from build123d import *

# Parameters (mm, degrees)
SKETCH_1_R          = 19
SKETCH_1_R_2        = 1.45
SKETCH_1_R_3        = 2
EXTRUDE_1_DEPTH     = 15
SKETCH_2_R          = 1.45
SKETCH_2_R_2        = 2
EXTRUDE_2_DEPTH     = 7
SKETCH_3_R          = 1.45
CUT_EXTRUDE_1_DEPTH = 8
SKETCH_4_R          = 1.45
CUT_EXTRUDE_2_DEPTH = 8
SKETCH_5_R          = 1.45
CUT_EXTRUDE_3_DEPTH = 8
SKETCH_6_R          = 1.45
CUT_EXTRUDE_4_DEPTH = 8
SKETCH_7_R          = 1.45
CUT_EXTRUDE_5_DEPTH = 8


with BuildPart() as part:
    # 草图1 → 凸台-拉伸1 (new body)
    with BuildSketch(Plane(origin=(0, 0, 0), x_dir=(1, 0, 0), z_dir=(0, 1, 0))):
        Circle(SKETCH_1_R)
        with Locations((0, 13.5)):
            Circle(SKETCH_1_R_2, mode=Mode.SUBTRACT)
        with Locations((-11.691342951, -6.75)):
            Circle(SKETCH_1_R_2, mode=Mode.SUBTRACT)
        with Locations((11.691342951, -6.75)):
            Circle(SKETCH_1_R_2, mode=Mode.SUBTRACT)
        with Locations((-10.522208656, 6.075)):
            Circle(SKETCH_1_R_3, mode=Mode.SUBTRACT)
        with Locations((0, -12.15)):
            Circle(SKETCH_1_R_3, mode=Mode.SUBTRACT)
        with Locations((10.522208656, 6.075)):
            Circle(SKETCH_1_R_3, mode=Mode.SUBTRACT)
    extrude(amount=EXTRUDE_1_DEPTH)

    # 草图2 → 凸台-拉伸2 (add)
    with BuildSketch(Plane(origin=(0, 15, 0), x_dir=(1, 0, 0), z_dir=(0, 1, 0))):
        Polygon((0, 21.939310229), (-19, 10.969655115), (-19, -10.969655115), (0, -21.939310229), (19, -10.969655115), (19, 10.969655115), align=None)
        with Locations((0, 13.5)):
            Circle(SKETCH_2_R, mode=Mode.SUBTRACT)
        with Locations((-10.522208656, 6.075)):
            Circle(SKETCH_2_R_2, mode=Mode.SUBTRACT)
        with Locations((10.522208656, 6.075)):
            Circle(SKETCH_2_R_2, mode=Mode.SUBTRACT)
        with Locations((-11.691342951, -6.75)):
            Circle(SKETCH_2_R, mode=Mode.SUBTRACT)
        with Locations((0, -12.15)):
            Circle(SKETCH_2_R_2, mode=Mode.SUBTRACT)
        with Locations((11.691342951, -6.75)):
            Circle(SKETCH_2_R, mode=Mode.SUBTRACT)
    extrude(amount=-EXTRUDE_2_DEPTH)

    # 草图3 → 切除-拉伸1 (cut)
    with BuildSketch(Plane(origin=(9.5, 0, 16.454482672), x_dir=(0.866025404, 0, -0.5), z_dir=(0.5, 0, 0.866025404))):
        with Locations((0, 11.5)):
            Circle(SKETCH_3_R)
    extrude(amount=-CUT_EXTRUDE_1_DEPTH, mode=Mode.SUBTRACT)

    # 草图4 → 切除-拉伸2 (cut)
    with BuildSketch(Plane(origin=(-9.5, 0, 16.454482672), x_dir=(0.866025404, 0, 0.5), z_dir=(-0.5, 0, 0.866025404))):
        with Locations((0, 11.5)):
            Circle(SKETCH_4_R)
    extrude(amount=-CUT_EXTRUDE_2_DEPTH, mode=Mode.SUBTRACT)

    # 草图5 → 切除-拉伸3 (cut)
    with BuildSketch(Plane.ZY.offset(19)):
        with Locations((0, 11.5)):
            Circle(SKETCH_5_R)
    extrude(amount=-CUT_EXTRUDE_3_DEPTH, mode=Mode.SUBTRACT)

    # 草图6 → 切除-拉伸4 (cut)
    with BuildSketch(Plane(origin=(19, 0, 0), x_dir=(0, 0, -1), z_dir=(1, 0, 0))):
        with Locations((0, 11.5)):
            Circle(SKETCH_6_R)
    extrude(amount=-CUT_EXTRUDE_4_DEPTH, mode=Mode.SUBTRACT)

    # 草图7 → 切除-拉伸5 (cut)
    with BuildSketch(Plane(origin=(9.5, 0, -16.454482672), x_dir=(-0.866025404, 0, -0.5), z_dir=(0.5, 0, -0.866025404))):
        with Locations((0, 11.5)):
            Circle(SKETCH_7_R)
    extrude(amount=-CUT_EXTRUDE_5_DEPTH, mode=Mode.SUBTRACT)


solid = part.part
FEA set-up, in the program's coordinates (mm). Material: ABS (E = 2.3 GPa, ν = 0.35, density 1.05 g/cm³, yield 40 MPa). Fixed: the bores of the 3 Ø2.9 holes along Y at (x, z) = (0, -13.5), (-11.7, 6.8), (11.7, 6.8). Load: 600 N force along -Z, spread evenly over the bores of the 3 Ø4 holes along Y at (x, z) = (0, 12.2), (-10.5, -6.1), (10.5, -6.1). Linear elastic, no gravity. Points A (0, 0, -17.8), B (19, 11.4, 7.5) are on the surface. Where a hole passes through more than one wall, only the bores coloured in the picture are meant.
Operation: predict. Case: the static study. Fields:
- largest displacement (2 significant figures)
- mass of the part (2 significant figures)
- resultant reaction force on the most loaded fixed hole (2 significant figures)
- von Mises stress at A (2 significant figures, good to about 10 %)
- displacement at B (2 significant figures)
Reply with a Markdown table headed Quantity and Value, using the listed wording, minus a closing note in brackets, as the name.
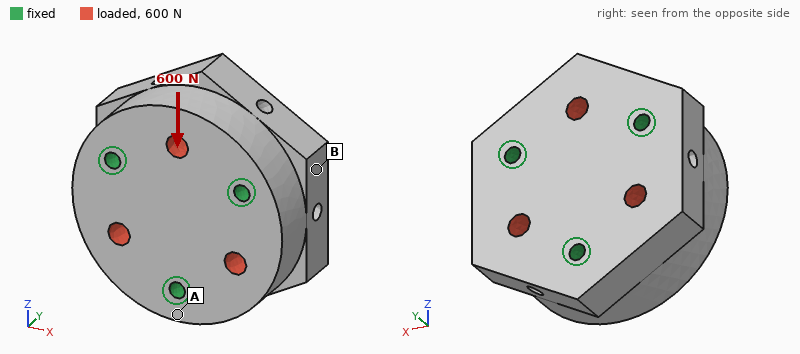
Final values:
| Quantity | Value |
|---|---|
| largest displacement | 8.4 µm |
| mass of the part | 18 g |
| resultant reaction force on the most loaded fixed hole | 210 N |
| von Mises stress at A | 0.79 MPa |
| displacement at B | 2.0 µm |
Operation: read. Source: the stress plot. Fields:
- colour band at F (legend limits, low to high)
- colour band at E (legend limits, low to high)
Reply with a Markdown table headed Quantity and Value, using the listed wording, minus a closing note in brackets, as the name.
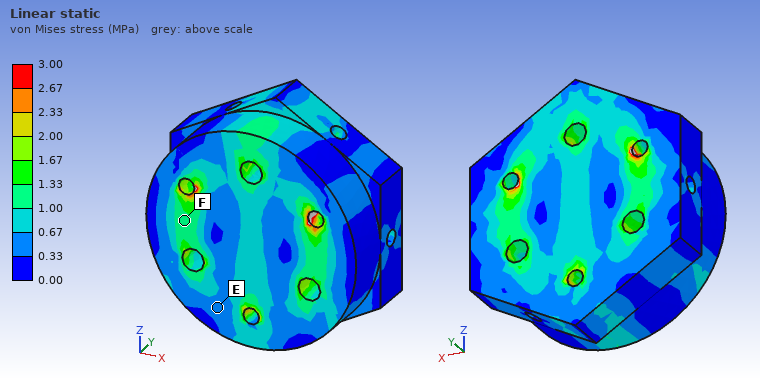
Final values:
| Quantity | Value |
|---|---|
| colour band at F | 1.00 to 1.33 MPa |
| colour band at E | 0.33 to 0.67 MPa |
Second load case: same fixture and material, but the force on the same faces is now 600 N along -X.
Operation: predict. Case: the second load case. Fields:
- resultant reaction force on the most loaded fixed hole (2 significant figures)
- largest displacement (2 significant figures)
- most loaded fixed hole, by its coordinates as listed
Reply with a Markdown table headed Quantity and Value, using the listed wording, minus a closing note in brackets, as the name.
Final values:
| Quantity | Value |
|---|---|
| resultant reaction force on the most loaded fixed hole | 220 N |
| largest displacement | 8.2 µm |
| most loaded fixed hole, by its coordinates as listed | (0, -13.5) |
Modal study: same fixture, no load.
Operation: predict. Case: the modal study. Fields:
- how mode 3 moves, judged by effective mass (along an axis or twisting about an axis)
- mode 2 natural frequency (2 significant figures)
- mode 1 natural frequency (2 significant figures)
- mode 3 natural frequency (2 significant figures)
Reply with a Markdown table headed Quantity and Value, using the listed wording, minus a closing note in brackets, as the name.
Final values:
| Quantity | Value |
|---|---|
| how mode 3 moves, judged by effective mass | along Y |
| mode 2 natural frequency | 11 kHz |
| mode 1 natural frequency | 11 kHz |
| mode 3 natural frequency | 12 kHz |
